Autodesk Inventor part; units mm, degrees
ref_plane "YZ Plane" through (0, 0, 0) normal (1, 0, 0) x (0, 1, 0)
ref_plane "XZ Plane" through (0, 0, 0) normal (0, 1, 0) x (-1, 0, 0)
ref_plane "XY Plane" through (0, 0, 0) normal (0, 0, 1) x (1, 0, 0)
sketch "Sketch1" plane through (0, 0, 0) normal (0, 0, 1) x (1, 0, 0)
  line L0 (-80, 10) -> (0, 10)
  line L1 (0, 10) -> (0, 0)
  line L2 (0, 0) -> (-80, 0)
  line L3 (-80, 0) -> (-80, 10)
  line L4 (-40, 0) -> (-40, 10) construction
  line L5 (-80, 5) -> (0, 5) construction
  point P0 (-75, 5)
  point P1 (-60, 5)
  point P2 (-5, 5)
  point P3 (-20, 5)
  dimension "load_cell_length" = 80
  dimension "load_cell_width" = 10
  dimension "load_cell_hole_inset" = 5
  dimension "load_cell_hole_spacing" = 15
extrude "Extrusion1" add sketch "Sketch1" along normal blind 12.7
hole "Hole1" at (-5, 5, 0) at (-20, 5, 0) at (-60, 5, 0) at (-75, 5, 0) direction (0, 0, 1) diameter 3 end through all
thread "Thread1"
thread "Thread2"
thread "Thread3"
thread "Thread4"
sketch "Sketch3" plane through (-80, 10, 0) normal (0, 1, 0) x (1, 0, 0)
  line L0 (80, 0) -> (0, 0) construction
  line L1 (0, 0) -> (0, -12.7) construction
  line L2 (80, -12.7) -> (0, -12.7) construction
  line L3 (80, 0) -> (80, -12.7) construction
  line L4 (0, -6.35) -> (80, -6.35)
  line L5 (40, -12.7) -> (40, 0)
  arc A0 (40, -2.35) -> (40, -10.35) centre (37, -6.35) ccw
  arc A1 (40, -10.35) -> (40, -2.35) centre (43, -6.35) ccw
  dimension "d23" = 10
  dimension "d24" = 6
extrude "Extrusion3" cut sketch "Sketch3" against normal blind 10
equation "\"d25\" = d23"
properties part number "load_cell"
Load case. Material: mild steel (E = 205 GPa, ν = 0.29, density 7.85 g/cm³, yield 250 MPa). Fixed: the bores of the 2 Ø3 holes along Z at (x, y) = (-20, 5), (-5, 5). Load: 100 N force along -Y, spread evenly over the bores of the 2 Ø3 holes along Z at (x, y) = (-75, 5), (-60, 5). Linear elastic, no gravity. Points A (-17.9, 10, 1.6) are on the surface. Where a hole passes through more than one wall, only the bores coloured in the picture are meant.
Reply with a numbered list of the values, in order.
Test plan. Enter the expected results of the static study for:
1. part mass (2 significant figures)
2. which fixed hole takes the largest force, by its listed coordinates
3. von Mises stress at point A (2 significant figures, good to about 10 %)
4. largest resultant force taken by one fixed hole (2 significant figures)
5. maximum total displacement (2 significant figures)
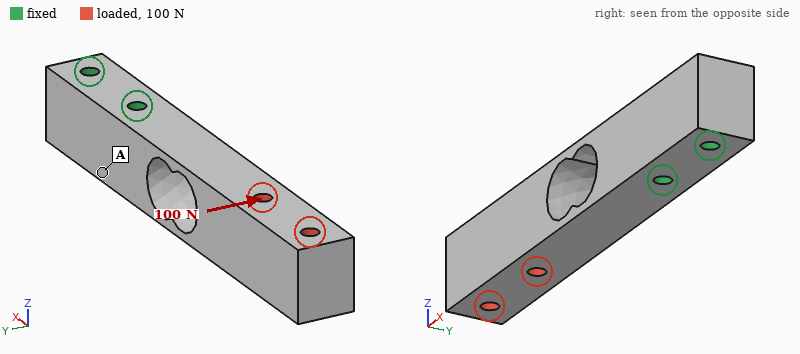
1. 66 g
2. (-20, 5)
3. 11 MPa
4. 270 N
5. 57 µm
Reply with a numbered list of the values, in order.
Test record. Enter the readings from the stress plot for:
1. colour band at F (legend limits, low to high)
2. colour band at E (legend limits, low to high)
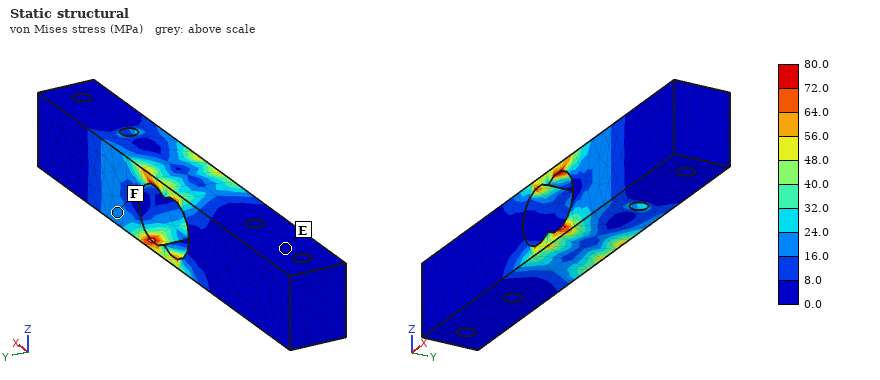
1. 16.0 to 24.0 MPa
2. 0.0 to 8.0 MPa
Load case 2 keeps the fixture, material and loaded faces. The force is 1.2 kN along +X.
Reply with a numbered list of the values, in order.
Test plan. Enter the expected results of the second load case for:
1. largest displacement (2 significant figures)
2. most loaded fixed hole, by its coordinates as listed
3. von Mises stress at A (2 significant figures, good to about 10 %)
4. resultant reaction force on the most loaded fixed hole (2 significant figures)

1. 5.4 µm
2. (-20, 5)
3. 4.3 MPa
4. 1.1 kN
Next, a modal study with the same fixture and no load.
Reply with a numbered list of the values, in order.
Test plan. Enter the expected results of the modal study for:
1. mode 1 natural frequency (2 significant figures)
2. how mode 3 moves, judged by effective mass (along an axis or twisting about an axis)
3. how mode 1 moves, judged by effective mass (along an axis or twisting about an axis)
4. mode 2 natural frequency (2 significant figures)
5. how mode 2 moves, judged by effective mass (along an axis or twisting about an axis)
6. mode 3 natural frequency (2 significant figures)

1. 1500 Hz
2. twisting about X
3. along Y
4. 1800 Hz
5. along Z
6. 7200 Hz
